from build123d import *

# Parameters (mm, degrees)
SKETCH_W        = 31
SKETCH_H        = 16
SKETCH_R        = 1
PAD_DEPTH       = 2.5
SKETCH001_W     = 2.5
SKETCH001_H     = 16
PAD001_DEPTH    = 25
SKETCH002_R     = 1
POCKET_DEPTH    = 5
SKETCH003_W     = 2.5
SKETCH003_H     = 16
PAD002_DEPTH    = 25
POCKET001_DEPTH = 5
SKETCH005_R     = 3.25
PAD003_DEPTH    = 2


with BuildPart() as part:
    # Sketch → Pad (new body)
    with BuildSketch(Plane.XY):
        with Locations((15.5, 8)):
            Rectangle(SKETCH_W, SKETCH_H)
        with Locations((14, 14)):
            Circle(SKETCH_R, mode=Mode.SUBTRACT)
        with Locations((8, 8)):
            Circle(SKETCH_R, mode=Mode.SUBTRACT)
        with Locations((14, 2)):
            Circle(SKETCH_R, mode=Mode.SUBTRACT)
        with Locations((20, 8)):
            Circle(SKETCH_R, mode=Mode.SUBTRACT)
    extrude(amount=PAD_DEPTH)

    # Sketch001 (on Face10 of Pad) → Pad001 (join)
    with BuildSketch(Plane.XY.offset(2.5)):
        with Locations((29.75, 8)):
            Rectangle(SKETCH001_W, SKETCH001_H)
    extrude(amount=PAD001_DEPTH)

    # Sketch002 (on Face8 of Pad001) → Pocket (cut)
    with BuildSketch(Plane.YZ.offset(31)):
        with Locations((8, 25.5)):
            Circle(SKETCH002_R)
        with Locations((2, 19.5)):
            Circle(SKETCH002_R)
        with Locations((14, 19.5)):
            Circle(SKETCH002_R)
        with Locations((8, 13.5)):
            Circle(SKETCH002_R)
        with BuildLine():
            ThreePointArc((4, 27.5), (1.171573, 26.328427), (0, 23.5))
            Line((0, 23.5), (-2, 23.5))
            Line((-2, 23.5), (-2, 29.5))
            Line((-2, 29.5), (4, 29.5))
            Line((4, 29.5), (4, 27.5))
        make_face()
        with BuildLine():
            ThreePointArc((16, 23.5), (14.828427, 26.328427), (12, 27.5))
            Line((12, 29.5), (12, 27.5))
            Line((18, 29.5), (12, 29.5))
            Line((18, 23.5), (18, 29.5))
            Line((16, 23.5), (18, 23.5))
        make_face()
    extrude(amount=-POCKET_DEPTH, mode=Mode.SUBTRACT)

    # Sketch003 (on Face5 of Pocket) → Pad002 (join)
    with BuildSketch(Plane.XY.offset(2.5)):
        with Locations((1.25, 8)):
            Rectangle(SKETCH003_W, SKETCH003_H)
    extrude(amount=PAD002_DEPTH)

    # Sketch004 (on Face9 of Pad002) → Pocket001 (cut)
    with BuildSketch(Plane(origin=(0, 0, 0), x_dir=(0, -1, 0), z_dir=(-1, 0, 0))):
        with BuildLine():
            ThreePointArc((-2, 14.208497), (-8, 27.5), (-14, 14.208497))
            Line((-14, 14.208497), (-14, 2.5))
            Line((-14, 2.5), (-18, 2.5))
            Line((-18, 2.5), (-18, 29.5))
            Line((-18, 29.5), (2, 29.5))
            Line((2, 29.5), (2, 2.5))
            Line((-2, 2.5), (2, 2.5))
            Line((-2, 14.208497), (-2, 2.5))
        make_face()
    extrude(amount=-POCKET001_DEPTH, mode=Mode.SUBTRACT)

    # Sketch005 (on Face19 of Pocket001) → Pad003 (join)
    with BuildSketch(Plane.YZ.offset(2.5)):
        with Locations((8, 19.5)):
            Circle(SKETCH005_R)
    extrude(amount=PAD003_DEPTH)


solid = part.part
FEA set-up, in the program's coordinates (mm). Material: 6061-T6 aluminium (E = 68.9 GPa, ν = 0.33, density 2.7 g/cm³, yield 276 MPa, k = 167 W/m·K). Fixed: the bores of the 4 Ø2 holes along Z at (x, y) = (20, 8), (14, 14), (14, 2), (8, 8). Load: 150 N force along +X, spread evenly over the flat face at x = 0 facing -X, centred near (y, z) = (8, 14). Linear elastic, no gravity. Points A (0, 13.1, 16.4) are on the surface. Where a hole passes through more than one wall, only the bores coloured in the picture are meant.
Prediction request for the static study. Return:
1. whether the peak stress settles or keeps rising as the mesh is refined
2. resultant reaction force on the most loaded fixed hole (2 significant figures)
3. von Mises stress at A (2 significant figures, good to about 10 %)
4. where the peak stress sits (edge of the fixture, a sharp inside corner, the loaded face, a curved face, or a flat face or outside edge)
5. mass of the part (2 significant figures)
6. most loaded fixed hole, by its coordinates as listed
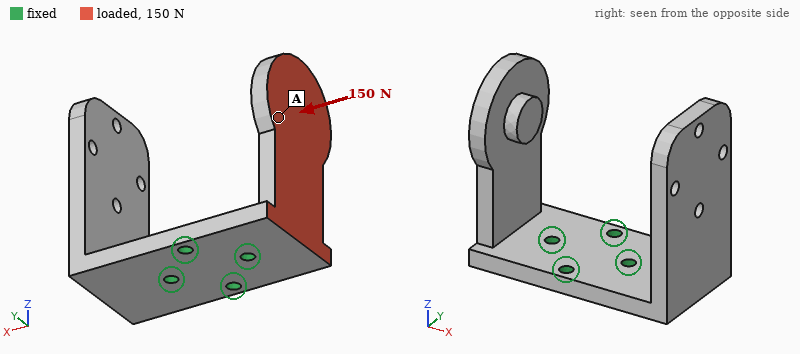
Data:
keeps rising
190 N
21 MPa
edge of the fixture
8.2 g
(8, 8)
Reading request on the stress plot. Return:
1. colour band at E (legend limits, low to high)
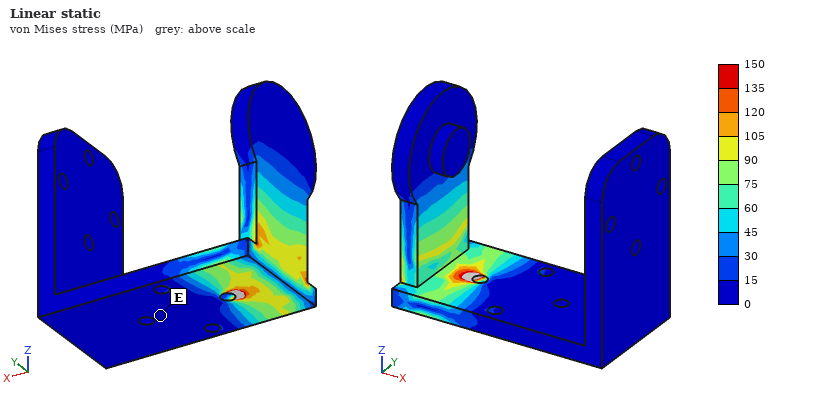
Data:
0 to 15 MPa
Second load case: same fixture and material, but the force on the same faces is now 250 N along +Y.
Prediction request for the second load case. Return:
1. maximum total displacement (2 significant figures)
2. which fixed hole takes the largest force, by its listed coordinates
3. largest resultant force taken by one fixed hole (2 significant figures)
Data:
0.24 mm
(8, 8)
270 N
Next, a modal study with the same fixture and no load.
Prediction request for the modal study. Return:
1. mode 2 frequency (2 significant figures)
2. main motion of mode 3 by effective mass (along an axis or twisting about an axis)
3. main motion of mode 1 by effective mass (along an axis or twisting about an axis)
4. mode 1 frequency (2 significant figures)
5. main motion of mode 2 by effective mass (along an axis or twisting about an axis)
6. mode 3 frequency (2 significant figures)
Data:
2100 Hz
along Y
along X
2000 Hz
along X
3100 Hz
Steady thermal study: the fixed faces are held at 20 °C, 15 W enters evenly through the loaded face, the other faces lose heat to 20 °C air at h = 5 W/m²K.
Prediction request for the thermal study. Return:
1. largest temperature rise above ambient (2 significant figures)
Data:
51 K
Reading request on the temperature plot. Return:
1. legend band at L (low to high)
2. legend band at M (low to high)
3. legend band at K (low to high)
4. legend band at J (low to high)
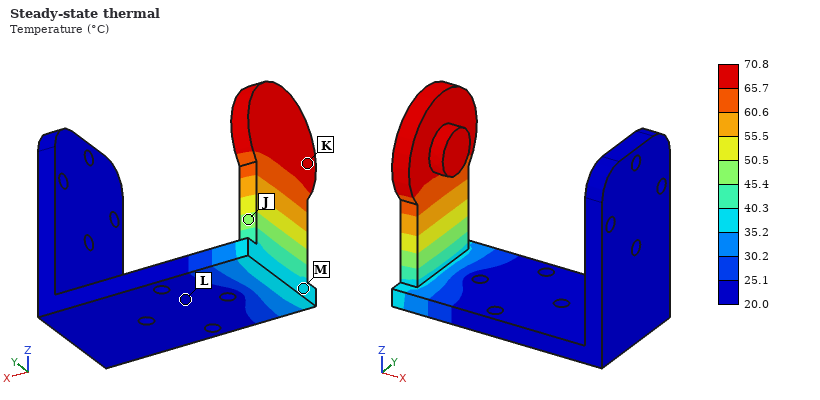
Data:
20.0 to 25.1 °C
35.2 to 40.3 °C
65.7 to 70.8 °C
45.4 to 50.5 °C
